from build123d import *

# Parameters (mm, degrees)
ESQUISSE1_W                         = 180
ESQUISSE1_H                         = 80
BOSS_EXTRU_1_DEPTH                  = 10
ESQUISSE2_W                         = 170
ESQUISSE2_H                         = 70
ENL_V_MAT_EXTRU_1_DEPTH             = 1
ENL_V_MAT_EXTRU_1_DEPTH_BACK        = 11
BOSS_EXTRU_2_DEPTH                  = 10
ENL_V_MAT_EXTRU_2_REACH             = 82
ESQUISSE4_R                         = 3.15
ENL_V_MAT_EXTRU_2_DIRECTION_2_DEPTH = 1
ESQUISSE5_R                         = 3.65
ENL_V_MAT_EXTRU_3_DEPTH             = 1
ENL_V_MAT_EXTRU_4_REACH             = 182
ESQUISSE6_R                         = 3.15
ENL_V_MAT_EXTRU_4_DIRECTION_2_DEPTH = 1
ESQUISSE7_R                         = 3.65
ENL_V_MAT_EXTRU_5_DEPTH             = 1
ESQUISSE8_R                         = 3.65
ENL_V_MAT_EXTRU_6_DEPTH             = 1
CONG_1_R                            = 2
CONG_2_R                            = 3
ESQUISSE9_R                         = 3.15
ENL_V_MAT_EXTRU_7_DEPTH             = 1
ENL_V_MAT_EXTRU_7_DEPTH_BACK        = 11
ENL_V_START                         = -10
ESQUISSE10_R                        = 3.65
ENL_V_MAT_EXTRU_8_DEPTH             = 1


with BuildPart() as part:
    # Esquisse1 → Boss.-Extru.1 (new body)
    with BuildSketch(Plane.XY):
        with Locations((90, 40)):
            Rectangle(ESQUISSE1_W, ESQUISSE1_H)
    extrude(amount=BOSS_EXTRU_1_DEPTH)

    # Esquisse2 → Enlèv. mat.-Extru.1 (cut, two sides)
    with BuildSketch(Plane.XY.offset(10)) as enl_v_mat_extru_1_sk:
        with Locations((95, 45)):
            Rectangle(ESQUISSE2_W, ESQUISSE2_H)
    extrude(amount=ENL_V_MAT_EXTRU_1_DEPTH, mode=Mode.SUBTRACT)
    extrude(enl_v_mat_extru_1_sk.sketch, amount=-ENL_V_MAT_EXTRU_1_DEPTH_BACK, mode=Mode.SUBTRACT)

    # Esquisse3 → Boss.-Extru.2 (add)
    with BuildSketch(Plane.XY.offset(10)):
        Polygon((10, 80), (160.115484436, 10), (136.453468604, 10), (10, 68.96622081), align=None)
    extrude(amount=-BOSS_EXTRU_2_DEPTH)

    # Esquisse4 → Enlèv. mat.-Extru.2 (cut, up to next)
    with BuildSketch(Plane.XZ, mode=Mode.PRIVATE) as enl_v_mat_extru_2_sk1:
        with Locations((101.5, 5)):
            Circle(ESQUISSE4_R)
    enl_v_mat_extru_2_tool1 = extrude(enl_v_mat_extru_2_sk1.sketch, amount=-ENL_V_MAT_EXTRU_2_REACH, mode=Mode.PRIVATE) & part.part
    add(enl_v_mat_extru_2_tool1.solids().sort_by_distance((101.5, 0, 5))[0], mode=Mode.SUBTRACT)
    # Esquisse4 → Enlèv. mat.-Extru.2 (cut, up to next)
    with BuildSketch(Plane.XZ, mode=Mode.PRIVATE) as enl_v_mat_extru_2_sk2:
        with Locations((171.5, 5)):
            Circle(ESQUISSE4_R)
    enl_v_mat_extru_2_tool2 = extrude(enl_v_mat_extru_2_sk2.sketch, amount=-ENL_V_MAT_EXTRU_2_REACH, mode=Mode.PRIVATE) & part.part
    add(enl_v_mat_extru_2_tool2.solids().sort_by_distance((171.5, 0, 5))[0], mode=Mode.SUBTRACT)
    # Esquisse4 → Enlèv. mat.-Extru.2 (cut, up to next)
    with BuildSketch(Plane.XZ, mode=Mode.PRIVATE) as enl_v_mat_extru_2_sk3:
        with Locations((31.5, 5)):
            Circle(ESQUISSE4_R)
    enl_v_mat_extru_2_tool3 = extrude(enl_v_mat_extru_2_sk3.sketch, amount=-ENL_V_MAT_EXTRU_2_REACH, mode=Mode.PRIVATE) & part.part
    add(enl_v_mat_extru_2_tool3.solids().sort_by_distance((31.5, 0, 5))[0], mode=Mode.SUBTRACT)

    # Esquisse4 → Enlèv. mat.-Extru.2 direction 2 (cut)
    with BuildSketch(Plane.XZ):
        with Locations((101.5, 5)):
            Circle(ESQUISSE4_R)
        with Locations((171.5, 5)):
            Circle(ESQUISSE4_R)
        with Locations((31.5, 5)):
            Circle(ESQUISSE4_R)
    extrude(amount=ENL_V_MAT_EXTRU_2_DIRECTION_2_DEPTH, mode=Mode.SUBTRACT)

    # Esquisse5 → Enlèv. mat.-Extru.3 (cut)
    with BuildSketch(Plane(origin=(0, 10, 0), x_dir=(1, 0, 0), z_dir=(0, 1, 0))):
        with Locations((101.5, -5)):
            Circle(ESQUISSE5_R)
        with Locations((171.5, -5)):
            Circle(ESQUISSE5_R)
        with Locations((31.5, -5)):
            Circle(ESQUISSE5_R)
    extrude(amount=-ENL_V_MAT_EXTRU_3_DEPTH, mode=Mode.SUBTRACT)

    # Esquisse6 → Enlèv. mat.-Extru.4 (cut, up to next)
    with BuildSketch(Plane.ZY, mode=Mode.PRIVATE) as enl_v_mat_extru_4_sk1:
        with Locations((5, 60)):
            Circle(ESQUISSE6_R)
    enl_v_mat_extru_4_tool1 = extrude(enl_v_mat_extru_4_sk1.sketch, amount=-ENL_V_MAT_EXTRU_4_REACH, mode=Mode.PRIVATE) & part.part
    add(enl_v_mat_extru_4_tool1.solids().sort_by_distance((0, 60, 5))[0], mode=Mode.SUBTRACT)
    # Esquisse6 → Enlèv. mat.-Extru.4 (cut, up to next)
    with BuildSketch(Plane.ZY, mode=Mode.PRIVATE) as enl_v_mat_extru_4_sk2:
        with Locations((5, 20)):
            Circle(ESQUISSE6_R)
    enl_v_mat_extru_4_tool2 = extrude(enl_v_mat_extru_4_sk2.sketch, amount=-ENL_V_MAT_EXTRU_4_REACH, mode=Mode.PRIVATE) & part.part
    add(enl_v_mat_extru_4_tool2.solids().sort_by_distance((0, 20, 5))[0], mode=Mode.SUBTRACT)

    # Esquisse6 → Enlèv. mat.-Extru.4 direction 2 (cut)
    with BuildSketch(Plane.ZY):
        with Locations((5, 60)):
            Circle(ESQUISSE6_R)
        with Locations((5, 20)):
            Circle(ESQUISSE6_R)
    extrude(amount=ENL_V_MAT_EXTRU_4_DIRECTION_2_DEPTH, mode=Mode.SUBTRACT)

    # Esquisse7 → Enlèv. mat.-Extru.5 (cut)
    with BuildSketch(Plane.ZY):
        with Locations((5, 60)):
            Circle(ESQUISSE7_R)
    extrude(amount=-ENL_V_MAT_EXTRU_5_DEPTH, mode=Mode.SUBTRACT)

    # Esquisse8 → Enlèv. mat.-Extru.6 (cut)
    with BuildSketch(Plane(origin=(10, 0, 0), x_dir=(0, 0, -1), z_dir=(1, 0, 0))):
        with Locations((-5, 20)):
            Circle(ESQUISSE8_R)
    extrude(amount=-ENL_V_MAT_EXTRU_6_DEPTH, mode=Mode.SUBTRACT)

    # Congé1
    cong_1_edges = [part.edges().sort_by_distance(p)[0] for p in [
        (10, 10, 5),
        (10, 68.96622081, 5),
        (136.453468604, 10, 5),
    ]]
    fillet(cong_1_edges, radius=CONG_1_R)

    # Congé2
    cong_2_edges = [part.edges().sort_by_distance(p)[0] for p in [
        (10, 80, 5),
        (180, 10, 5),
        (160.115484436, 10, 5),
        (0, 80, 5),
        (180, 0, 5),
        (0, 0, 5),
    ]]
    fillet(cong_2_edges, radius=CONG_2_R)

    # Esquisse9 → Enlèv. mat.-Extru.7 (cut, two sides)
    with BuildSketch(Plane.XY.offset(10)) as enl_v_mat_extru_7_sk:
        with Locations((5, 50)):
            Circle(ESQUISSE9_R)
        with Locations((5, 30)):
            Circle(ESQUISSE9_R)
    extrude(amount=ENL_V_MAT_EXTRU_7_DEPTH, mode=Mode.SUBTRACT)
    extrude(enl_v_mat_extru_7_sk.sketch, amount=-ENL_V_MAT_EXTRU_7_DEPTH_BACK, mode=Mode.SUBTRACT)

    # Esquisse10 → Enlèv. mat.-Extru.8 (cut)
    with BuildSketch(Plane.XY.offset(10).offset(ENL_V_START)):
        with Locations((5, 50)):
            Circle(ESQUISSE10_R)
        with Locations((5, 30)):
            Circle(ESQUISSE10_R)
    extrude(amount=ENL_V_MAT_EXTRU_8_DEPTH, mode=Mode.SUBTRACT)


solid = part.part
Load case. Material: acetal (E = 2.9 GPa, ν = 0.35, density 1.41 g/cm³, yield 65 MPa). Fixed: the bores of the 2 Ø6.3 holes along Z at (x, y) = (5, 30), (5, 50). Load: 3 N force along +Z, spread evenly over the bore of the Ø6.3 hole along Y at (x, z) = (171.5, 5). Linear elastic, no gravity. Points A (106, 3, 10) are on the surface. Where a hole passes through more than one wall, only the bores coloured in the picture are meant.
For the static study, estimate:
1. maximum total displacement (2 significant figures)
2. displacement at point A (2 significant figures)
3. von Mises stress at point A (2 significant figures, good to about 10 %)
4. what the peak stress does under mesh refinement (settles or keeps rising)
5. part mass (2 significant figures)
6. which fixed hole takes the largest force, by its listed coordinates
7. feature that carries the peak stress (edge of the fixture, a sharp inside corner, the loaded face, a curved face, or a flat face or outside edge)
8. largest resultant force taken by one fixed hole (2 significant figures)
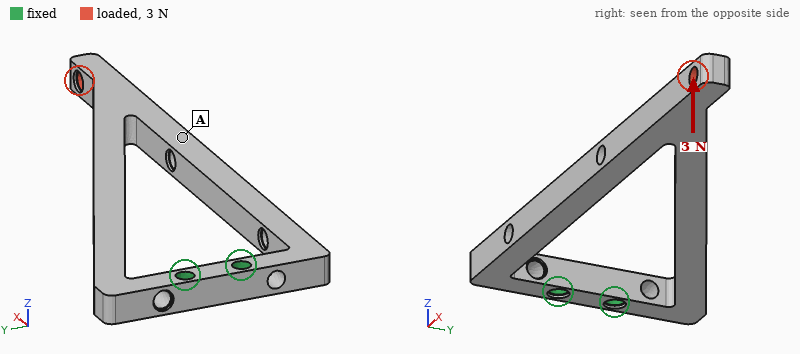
2.0 mm
0.99 mm
0.59 MPa
keeps rising
54 g
(5, 30)
edge of the fixture
1.9 N
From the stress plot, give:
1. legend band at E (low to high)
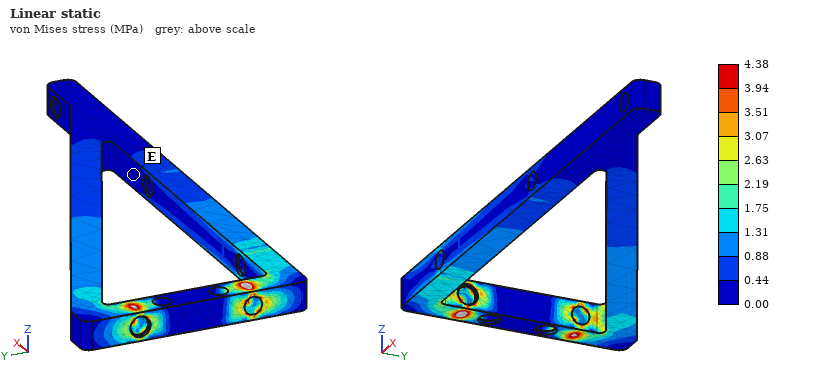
0.00 to 0.44 MPa
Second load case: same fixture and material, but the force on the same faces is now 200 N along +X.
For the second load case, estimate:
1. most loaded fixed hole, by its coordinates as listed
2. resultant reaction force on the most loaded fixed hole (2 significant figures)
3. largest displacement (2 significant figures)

(5, 30)
230 N
2.1 mm
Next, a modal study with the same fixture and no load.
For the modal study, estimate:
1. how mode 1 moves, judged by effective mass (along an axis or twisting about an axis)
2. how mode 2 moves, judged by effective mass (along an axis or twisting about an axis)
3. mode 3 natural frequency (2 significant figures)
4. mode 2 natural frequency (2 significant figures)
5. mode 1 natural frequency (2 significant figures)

along Z
along Y
380 Hz
160 Hz
59 Hz
